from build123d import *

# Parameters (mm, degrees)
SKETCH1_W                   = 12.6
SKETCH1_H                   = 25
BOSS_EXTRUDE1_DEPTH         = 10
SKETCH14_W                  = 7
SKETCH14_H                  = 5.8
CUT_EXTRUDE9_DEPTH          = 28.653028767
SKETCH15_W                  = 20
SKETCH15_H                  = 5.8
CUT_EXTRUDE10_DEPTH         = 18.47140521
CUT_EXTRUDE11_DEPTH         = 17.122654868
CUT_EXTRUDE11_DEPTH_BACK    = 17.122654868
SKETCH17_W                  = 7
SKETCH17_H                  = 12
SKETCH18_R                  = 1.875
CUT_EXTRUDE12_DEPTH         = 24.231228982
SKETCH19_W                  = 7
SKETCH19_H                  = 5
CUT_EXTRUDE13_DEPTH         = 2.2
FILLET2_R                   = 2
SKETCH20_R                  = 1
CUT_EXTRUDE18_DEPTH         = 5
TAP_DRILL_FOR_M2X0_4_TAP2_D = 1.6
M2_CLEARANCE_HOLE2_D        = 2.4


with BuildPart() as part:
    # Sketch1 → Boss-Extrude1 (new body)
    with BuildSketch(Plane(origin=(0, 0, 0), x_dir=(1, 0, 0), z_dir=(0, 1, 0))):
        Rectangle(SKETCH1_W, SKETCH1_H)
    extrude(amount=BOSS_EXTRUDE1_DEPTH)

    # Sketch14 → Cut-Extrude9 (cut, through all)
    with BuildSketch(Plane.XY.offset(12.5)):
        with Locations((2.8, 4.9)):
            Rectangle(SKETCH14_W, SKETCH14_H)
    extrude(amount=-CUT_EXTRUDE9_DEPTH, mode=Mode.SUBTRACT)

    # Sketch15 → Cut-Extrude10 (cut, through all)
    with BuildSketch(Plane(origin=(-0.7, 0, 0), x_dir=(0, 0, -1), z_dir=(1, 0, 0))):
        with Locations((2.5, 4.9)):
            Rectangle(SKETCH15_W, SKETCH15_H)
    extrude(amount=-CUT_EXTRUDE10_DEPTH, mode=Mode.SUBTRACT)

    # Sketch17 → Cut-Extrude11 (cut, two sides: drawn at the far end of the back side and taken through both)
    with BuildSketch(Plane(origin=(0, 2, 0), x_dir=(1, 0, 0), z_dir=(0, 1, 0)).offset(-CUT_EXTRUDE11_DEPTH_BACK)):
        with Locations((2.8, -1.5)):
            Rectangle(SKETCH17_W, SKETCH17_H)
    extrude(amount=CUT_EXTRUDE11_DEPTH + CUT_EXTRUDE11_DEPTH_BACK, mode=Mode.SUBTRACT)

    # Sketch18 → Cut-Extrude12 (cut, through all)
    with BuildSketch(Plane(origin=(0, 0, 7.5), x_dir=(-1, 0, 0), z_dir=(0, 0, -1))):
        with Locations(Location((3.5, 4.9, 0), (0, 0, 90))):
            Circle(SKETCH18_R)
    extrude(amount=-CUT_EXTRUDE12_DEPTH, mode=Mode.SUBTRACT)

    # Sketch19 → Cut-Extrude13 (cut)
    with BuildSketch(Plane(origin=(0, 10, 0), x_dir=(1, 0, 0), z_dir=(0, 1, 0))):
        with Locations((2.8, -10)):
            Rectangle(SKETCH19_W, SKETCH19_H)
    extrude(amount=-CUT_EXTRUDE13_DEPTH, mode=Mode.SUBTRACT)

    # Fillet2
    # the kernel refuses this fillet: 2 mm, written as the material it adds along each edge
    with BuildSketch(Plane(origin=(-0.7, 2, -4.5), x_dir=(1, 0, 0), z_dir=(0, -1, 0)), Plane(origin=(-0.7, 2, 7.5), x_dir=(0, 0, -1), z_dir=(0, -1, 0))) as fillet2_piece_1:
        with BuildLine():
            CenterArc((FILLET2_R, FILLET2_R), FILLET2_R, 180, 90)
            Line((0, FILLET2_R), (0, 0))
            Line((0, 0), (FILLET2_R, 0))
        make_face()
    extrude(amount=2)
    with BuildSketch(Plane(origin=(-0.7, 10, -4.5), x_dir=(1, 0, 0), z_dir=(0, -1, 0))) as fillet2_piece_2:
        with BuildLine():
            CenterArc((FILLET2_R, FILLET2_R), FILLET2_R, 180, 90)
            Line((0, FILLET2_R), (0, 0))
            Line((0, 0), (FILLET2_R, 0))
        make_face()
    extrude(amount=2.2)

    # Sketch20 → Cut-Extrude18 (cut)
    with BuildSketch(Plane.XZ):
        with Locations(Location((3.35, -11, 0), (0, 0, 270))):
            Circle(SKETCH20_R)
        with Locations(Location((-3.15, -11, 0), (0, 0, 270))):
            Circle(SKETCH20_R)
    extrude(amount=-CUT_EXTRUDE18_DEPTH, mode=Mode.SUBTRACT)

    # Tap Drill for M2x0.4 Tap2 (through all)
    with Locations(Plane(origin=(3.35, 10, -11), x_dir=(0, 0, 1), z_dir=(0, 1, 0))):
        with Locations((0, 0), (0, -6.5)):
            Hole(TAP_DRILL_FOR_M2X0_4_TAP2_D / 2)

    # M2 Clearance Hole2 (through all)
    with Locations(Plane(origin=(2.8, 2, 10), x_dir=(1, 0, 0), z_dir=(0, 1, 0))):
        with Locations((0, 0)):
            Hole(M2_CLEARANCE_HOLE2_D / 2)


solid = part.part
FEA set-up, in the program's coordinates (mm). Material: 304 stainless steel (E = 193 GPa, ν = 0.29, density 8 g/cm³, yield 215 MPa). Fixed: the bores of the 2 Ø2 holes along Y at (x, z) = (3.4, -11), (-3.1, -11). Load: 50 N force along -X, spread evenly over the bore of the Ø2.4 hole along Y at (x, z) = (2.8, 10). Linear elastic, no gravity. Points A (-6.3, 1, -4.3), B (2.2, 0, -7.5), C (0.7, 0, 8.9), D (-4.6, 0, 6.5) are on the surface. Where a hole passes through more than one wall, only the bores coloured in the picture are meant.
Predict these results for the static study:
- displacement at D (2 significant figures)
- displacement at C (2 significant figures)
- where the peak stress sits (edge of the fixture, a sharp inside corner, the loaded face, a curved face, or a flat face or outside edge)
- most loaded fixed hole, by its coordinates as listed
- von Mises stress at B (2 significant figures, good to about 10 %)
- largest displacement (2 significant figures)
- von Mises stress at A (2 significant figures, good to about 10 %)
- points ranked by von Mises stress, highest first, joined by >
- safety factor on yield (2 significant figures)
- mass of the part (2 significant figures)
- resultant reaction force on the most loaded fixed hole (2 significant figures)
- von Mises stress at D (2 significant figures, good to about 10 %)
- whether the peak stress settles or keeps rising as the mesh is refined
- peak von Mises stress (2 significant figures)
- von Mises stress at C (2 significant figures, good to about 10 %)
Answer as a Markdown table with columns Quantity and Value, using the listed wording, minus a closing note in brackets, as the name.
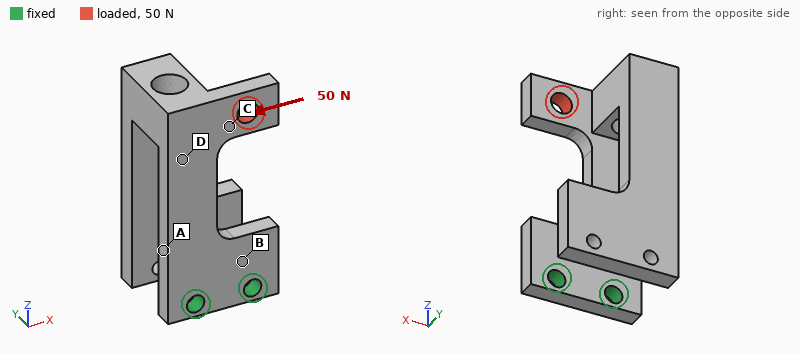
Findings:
| Quantity | Value |
|---|---|
| displacement at D | 11 µm |
| displacement at C | 15 µm |
| where the peak stress sits | a curved face |
| most loaded fixed hole, by its coordinates as listed | (3.4, -11) |
| von Mises stress at B | 20 MPa |
| largest displacement | 22 µm |
| von Mises stress at A | 54 MPa |
| points ranked by von Mises stress, highest first, joined by > | A > B > D > C |
| safety factor on yield | 2.3 |
| mass of the part | 7.8 g |
| resultant reaction force on the most loaded fixed hole | 150 N |
| von Mises stress at D | 12 MPa |
| whether the peak stress settles or keeps rising as the mesh is refined | settles |
| peak von Mises stress | 95 MPa |
| von Mises stress at C | 5.3 MPa |
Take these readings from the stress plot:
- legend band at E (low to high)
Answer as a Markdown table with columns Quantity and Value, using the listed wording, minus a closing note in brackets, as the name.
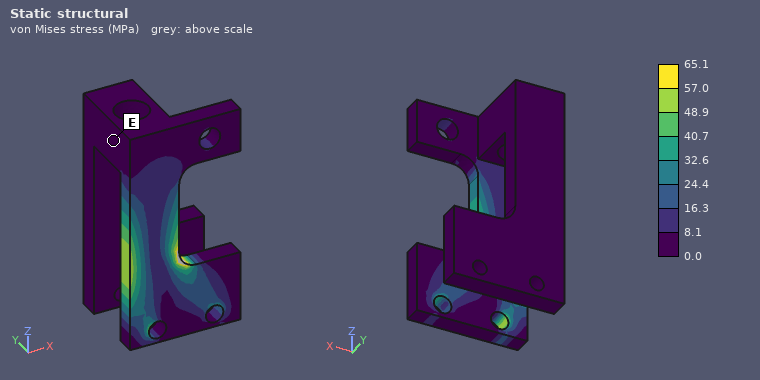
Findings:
| Quantity | Value |
|---|---|
| legend band at E | 0.0 to 8.1 MPa |
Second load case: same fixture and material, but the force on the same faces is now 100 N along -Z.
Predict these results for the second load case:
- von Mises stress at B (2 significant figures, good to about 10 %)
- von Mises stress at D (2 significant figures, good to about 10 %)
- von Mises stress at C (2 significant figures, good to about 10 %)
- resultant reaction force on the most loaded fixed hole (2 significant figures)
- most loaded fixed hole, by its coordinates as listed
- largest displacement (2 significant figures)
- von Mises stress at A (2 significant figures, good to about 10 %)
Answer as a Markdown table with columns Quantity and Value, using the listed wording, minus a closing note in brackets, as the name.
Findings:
| Quantity | Value |
|---|---|
| von Mises stress at B | 13 MPa |
| von Mises stress at D | 19 MPa |
| von Mises stress at C | 28 MPa |
| resultant reaction force on the most loaded fixed hole | 92 N |
| most loaded fixed hole, by its coordinates as listed | (3.4, -11) |
| largest displacement | 28 µm |
| von Mises stress at A | 40 MPa |
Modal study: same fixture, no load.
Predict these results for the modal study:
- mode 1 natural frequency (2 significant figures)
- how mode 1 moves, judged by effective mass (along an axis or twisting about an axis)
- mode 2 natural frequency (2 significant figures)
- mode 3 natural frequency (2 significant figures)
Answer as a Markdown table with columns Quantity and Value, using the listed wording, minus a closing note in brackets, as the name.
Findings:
| Quantity | Value |
|---|---|
| mode 1 natural frequency | 1300 Hz |
| how mode 1 moves, judged by effective mass | along Z |
| mode 2 natural frequency | 1800 Hz |
| mode 3 natural frequency | 2100 Hz |
